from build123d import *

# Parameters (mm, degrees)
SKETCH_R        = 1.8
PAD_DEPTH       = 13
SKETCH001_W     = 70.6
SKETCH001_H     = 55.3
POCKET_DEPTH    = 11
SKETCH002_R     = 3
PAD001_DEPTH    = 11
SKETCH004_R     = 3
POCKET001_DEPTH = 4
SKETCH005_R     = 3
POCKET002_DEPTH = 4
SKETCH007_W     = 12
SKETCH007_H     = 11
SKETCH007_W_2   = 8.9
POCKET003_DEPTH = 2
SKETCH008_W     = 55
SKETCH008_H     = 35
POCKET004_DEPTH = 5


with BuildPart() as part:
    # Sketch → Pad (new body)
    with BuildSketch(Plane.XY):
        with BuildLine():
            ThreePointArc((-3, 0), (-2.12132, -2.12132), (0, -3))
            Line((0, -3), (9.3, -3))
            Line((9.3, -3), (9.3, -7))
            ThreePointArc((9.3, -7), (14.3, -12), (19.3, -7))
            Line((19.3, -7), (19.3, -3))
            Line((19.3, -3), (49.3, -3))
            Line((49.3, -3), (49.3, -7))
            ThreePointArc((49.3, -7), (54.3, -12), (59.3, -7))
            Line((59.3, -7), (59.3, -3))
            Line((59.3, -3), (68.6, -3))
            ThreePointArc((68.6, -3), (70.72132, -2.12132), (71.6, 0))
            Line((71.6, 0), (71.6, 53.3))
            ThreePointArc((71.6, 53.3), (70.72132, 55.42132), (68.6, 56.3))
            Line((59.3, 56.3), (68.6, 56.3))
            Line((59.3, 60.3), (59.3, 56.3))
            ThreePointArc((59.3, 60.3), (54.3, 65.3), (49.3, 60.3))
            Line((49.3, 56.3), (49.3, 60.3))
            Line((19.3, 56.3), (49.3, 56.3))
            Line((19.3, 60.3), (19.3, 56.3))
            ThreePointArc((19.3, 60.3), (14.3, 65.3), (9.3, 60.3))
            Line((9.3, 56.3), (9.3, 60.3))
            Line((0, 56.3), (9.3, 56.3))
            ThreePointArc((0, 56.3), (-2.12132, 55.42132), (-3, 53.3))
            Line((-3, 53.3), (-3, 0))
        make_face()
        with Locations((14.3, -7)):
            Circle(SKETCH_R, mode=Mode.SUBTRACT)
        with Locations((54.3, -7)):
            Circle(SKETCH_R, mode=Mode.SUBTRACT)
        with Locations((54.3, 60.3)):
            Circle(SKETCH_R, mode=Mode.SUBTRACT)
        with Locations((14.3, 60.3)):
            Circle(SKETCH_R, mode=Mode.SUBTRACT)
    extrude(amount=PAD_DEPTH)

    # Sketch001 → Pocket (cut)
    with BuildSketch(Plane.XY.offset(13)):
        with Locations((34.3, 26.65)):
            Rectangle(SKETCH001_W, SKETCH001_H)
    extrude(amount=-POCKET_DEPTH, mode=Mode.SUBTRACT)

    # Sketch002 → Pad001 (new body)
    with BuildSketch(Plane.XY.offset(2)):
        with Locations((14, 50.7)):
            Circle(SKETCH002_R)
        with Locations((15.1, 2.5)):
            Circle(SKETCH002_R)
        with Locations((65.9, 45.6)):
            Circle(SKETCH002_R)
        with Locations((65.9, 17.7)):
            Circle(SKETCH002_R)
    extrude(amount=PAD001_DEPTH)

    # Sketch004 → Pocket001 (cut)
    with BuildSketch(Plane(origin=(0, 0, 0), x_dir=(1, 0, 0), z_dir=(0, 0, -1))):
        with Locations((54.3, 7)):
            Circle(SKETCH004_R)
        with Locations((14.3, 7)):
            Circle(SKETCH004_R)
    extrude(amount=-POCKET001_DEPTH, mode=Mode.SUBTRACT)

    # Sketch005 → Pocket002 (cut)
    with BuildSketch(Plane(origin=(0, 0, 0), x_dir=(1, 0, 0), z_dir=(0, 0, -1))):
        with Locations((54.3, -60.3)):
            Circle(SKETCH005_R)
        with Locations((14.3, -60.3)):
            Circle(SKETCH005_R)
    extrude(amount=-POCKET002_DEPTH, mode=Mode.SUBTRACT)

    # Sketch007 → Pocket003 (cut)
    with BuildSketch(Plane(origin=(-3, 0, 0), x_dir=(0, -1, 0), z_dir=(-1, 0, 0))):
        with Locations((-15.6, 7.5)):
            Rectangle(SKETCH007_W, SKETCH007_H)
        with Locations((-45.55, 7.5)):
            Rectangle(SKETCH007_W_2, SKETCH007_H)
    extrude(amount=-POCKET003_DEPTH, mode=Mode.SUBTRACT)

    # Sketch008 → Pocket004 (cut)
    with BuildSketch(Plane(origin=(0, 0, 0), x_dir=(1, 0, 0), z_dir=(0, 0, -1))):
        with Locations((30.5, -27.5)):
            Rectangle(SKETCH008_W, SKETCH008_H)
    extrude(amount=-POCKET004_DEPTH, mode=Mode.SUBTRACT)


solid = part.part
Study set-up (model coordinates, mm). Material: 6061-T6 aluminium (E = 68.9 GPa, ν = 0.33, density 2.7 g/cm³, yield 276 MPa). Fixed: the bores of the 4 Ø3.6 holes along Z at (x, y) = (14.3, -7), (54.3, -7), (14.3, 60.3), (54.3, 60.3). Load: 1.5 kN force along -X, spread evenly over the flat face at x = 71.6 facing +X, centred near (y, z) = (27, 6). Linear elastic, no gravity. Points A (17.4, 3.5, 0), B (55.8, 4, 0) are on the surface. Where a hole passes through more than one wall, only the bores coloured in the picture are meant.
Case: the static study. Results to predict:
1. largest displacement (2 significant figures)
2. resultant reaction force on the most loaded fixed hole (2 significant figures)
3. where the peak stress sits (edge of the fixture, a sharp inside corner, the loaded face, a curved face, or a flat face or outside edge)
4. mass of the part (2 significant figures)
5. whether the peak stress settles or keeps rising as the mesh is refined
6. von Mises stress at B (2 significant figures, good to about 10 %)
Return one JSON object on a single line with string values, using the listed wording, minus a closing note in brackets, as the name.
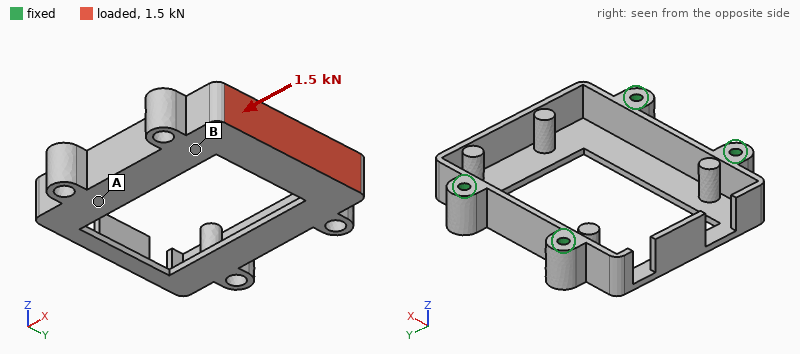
{"largest displacement": "0.35 mm", "resultant reaction force on the most loaded fixed hole": "690 N", "where the peak stress sits": "a sharp inside corner", "mass of the part": "40 g", "whether the peak stress settles or keeps rising as the mesh is refined": "keeps rising", "von Mises stress at B": "57 MPa"}
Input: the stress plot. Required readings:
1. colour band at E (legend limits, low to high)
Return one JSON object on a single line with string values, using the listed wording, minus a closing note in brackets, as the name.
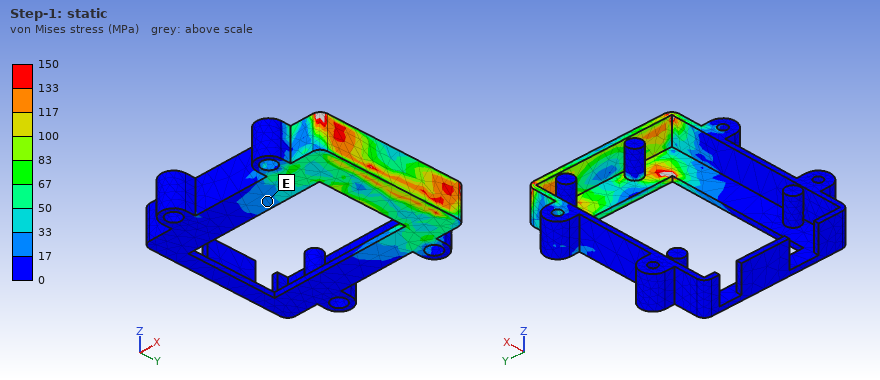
{"colour band at E": "17 to 33 MPa"}
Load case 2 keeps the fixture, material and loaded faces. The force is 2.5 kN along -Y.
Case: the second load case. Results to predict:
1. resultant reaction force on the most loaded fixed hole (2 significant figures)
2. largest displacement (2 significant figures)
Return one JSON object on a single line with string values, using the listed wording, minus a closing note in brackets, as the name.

{"resultant reaction force on the most loaded fixed hole": "1.4 kN", "largest displacement": "67 µm"}
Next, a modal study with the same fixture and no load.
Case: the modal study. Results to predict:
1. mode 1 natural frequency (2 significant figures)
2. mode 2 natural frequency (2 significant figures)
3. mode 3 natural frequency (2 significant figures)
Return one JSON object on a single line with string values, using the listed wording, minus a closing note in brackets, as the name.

{"mode 1 natural frequency": "3500 Hz", "mode 2 natural frequency": "4200 Hz", "mode 3 natural frequency": "5200 Hz"}
